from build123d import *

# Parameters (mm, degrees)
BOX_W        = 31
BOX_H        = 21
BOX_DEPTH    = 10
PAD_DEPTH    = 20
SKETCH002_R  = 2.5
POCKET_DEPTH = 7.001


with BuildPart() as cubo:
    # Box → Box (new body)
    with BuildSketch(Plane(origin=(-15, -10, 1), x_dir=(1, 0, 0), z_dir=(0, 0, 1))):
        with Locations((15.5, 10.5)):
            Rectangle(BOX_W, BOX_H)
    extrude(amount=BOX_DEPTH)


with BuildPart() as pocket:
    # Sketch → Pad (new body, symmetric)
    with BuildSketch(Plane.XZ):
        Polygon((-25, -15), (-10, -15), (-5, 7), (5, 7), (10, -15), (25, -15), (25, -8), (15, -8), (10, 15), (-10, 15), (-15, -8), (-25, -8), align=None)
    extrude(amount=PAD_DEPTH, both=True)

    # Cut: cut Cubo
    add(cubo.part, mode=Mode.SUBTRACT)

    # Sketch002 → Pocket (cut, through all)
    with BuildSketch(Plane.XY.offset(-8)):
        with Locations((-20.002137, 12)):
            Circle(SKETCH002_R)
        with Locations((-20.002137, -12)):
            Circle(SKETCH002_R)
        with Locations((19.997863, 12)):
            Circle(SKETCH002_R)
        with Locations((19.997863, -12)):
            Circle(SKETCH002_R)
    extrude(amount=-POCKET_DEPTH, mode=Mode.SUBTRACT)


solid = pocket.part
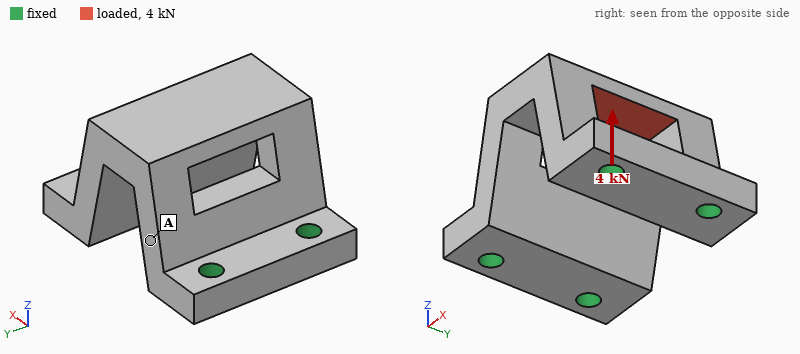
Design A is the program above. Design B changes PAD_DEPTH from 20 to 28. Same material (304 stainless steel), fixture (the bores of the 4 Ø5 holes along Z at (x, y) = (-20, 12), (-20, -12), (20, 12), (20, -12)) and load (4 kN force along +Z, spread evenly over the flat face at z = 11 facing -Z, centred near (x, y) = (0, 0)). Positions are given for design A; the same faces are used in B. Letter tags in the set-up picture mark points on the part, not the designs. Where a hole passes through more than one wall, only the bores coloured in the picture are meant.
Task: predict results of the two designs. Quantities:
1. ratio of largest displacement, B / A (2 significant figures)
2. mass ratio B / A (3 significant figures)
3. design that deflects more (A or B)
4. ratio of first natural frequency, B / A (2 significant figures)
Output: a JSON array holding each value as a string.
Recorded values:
["0.91", "1.48", "A", "0.85"]
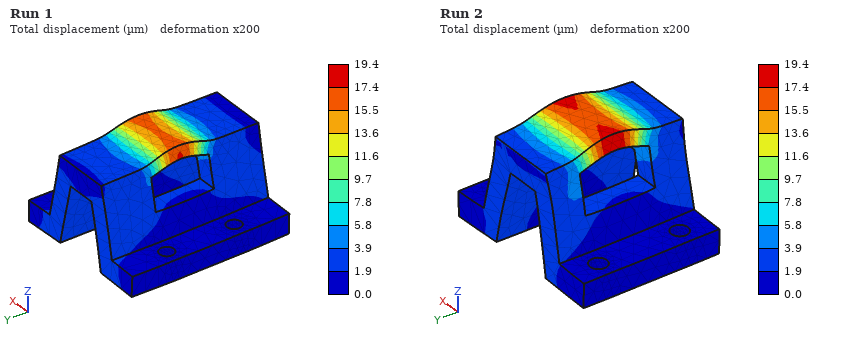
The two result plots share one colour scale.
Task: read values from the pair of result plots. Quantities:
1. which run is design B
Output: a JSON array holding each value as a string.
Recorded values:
["Run 1"]
